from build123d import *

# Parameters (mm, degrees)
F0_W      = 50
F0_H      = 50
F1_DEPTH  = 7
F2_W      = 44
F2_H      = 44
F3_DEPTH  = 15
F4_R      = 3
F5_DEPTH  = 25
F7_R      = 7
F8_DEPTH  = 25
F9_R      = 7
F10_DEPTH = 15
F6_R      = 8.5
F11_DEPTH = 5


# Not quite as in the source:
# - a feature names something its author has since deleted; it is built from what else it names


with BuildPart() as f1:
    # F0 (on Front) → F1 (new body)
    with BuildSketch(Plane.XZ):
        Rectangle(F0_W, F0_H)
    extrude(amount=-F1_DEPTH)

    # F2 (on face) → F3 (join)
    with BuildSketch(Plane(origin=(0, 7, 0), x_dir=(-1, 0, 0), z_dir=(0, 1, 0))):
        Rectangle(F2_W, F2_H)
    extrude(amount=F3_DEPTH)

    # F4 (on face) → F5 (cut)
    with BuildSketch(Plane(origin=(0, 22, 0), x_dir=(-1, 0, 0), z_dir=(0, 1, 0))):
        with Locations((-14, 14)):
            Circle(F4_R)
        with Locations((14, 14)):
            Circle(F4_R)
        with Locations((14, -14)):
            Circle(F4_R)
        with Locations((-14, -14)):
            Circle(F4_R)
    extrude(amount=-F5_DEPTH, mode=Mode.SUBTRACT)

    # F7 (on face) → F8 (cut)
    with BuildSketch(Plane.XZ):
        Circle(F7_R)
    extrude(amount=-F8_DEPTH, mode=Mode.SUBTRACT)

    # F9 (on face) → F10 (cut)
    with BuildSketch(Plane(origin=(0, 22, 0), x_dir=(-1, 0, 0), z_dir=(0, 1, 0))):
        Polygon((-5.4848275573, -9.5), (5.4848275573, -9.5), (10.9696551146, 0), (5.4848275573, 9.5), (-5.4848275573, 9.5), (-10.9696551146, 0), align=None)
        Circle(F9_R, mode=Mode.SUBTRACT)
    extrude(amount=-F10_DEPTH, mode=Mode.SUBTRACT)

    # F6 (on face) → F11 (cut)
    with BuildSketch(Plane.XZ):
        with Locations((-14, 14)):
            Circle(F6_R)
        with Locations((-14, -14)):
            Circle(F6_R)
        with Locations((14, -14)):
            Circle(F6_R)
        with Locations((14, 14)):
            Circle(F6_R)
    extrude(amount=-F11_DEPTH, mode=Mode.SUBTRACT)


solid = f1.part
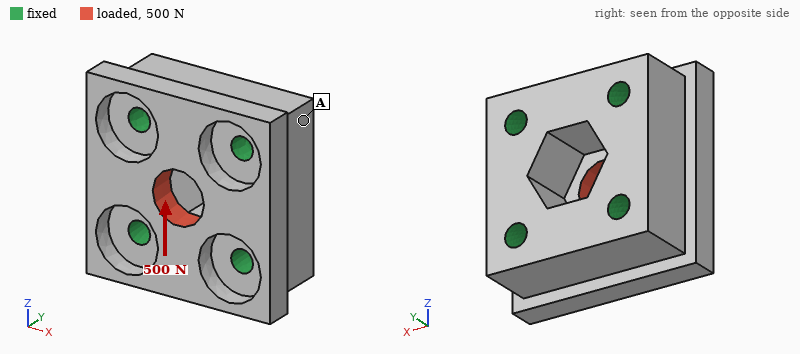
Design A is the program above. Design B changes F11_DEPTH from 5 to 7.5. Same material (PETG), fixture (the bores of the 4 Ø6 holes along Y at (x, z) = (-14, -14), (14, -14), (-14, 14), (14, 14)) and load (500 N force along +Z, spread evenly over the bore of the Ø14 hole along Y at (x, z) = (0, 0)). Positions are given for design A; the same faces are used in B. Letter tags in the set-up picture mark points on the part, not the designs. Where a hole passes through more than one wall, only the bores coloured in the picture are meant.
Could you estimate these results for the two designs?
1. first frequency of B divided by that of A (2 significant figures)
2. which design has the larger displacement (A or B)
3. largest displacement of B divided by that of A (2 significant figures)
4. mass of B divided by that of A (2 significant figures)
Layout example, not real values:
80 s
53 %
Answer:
0.81
B
1.3
0.94
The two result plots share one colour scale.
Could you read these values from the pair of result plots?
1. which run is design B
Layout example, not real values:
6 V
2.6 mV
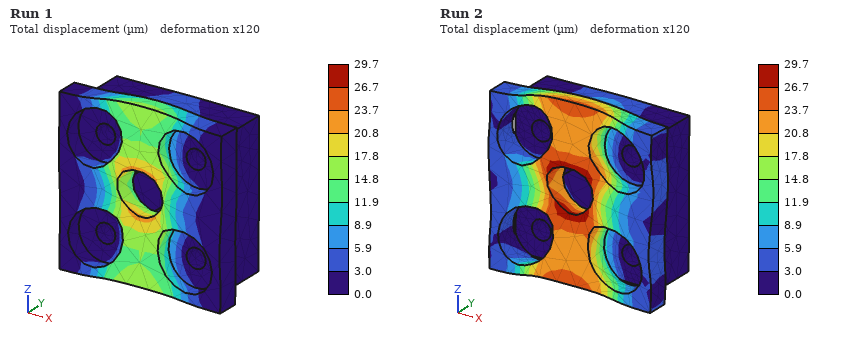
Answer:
Run 2
